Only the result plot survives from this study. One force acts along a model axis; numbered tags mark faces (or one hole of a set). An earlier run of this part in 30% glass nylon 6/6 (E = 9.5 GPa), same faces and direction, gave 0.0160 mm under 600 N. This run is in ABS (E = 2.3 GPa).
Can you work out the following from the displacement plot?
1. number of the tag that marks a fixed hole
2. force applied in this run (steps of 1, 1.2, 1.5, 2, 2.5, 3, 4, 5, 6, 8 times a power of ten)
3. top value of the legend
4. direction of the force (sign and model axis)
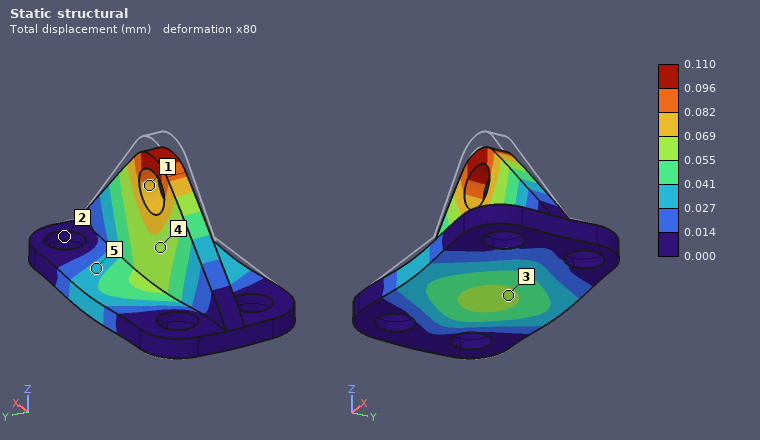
2
1 kN
0.110 mm
-Z
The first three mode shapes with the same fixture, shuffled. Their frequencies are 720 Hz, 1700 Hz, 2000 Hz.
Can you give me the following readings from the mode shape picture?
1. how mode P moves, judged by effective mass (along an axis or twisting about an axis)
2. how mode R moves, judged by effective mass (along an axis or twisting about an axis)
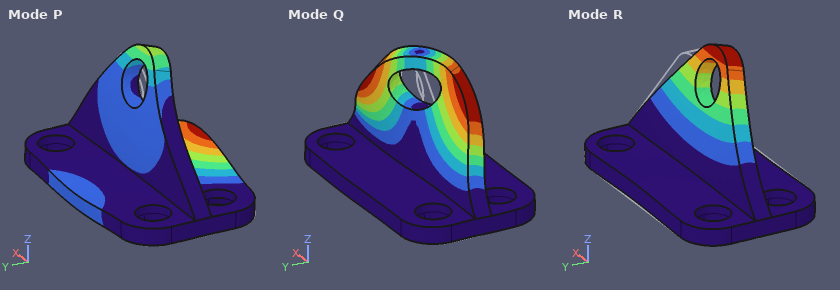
along Z
along Y
